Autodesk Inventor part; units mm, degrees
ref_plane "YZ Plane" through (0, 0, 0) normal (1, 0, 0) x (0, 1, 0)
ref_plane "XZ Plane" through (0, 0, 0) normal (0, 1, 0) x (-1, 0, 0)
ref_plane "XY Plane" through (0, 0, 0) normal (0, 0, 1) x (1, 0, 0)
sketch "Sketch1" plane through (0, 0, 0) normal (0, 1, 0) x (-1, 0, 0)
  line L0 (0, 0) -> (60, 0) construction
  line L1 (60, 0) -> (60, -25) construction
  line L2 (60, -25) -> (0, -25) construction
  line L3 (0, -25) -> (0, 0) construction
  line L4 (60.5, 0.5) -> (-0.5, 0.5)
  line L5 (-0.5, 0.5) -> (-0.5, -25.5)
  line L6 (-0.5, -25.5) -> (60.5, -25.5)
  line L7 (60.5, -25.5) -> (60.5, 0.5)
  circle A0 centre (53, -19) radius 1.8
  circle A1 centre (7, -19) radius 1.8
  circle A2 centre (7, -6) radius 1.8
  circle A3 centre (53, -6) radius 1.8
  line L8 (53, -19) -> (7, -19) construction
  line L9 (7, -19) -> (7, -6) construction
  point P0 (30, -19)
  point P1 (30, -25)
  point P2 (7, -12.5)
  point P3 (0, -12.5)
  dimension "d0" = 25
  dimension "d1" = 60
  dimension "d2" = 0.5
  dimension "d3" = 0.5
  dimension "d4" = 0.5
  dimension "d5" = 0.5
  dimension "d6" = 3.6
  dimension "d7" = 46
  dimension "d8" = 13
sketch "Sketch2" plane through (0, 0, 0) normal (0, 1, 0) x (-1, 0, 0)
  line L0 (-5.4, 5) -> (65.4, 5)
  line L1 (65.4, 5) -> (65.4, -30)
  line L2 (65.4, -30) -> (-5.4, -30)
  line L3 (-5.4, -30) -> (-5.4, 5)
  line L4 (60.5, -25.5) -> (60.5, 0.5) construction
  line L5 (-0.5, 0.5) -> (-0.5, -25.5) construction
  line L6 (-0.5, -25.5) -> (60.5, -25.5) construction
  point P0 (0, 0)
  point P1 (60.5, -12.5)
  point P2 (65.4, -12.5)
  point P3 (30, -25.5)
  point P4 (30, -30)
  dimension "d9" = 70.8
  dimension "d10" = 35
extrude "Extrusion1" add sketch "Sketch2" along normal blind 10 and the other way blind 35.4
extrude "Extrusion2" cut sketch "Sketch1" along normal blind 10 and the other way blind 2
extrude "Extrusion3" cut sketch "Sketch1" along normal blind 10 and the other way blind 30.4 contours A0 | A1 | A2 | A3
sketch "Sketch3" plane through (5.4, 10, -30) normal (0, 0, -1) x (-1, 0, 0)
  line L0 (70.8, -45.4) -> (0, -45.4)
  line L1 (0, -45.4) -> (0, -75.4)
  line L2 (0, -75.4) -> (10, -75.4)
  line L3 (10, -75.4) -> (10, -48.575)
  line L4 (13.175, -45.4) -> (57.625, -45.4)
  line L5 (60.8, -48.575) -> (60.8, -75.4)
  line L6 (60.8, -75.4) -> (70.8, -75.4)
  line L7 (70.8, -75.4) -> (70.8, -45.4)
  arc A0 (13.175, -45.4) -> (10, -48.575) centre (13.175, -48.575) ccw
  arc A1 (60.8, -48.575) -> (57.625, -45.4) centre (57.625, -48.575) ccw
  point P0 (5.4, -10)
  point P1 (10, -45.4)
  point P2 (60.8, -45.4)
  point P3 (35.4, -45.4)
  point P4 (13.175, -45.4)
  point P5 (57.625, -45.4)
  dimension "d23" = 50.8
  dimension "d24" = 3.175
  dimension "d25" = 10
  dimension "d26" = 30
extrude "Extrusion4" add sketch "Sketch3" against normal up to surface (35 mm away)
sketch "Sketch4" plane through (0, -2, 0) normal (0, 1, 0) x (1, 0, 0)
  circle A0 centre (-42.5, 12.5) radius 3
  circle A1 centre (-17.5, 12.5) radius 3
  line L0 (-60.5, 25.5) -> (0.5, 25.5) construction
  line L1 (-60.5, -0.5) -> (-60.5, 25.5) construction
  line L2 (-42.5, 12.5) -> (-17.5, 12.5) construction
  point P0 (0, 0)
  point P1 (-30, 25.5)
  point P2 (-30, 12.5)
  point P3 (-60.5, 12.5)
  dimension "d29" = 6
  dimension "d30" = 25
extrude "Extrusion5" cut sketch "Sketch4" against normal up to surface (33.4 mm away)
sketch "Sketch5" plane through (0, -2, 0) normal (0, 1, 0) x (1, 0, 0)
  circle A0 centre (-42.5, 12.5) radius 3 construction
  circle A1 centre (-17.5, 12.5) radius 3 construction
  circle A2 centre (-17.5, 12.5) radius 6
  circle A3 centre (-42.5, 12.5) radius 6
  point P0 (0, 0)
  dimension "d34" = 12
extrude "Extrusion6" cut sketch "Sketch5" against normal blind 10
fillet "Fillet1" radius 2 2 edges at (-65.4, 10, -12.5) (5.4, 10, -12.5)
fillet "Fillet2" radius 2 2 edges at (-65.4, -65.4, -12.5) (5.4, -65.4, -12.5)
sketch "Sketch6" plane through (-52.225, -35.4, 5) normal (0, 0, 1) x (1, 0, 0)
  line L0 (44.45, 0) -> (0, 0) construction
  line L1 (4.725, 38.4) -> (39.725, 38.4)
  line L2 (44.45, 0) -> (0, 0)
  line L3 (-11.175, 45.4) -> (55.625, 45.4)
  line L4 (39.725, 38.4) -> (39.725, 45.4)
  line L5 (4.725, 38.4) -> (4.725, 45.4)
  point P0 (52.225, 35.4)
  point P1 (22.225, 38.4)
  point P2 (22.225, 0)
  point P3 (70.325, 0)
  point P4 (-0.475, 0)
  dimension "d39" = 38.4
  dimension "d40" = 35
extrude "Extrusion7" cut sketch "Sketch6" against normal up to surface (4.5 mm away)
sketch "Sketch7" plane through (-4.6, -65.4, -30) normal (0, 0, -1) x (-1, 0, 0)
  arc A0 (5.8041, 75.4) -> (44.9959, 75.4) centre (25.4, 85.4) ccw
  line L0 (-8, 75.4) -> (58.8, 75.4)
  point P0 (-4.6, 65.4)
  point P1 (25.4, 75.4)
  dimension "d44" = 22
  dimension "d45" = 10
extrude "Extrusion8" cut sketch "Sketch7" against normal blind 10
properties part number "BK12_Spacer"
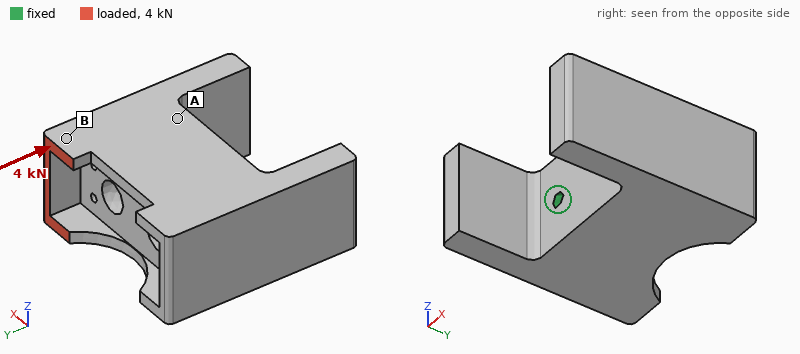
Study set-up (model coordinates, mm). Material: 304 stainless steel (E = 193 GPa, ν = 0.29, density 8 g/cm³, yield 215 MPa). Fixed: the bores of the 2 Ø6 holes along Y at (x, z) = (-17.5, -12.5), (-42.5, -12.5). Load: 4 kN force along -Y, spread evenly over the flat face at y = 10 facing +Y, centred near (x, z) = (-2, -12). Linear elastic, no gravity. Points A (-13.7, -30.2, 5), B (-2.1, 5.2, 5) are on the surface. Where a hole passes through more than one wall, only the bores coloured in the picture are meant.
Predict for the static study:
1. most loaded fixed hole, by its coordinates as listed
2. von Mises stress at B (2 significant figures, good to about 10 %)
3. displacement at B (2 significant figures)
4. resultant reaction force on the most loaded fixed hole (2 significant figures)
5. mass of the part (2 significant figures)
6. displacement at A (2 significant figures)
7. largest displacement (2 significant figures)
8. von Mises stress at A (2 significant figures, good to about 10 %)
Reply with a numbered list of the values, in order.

1. (-17.5, -12.5)
2. 19 MPa
3. 4.3 µm
4. 4.6 kN
5. 860 g
6. 1.0 µm
7. 5.0 µm
8. 3.3 MPa
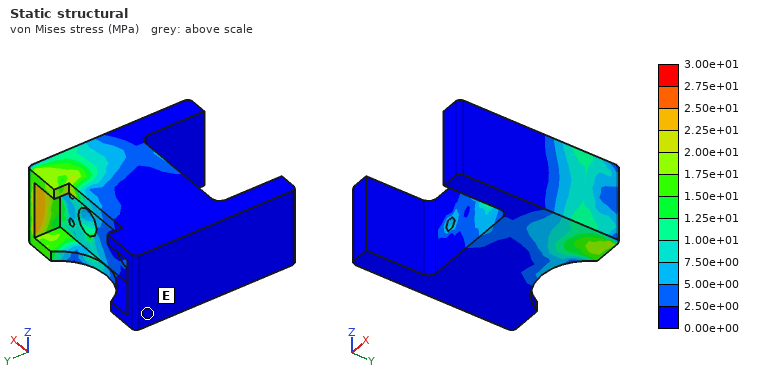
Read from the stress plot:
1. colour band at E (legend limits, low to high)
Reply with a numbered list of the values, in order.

1. 0.00e+00 to 2.50e+00 MPa
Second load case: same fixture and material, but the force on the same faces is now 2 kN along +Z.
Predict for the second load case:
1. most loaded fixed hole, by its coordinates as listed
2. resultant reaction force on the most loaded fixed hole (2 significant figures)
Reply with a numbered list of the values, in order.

1. (-17.5, -12.5)
2. 2.9 kN
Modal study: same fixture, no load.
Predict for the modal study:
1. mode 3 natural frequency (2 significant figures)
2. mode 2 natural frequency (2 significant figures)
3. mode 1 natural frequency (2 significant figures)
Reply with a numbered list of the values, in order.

1. 7700 Hz
2. 6100 Hz
3. 5900 Hz
